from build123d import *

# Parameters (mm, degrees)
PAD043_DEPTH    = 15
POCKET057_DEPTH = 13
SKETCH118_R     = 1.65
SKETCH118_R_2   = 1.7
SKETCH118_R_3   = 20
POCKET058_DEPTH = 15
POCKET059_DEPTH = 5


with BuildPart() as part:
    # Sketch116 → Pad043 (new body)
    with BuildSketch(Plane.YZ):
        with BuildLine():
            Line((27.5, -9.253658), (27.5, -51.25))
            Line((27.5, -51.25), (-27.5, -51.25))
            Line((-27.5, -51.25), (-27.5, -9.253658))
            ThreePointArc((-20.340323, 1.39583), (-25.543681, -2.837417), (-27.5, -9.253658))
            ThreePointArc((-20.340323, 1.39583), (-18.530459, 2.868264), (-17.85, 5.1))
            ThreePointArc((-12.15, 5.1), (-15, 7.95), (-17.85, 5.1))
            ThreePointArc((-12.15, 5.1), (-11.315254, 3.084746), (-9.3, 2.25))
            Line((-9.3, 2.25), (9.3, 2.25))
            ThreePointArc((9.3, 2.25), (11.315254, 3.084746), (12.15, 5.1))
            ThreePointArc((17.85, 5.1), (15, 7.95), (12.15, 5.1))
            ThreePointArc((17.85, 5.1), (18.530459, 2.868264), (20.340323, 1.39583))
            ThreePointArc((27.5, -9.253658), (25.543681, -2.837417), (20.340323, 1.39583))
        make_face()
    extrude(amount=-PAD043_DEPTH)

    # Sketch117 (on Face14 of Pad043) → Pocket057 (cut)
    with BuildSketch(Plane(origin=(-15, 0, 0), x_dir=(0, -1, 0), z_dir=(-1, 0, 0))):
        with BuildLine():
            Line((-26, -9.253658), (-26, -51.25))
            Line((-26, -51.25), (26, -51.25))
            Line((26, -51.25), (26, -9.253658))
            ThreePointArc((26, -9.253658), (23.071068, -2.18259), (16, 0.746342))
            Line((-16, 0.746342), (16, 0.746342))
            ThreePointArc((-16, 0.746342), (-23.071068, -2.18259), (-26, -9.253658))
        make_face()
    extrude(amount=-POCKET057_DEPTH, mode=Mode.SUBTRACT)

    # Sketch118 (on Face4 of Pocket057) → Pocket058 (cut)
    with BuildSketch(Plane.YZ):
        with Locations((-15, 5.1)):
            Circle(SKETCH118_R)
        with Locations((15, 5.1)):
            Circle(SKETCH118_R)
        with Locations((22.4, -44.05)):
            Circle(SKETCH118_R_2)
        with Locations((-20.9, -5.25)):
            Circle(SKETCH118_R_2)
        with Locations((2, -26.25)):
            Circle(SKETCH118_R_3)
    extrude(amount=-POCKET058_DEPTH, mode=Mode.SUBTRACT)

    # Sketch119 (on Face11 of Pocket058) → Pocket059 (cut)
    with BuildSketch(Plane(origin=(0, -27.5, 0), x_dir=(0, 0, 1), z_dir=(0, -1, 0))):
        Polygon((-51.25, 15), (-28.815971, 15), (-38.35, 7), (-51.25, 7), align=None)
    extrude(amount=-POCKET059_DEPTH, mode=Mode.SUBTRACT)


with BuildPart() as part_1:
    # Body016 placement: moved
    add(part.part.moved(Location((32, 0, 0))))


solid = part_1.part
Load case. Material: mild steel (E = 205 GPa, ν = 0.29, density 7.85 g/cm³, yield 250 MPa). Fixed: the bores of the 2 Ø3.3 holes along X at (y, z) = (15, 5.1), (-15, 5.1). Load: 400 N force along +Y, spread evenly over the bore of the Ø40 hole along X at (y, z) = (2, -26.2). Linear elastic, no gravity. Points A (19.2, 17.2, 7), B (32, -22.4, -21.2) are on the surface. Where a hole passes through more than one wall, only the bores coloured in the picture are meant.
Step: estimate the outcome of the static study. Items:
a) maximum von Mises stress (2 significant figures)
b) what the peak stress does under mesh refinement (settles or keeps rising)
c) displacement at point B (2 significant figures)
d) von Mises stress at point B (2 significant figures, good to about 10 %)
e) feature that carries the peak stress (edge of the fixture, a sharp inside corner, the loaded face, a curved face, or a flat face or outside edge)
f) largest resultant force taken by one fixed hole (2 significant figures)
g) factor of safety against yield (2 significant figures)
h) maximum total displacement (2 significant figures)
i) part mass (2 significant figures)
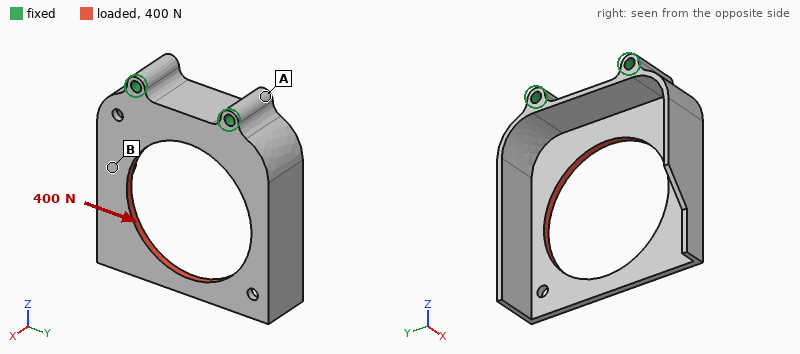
64 MPa
settles
14 µm
12 MPa
the loaded face
390 N
3.9
44 µm
52 g
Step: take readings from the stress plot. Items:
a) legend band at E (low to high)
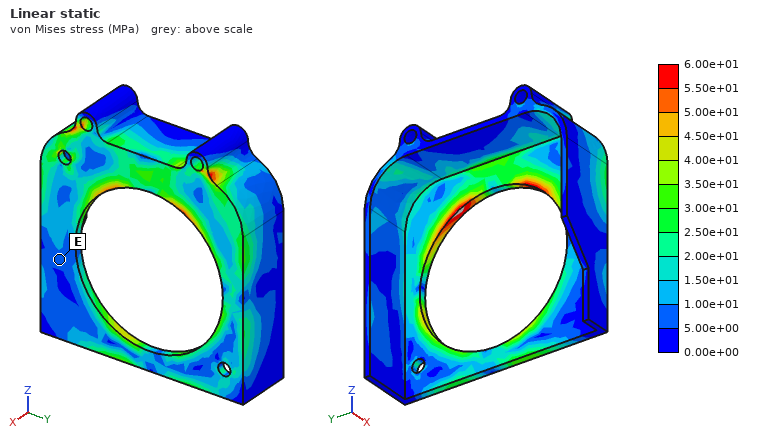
5.00e+00 to 1.00e+01 MPa
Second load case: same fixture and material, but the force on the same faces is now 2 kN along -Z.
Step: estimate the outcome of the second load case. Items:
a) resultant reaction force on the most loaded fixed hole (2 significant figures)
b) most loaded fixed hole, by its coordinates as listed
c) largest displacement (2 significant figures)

1.1 kN
(15, 5.1)
54 µm
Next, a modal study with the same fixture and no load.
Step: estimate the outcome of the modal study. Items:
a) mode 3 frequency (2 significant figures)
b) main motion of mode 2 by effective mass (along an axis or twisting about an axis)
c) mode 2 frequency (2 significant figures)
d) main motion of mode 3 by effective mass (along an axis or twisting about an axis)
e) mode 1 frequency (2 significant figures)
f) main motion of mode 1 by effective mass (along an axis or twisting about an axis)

2800 Hz
twisting about Z
1800 Hz
along Y
1200 Hz
along X
